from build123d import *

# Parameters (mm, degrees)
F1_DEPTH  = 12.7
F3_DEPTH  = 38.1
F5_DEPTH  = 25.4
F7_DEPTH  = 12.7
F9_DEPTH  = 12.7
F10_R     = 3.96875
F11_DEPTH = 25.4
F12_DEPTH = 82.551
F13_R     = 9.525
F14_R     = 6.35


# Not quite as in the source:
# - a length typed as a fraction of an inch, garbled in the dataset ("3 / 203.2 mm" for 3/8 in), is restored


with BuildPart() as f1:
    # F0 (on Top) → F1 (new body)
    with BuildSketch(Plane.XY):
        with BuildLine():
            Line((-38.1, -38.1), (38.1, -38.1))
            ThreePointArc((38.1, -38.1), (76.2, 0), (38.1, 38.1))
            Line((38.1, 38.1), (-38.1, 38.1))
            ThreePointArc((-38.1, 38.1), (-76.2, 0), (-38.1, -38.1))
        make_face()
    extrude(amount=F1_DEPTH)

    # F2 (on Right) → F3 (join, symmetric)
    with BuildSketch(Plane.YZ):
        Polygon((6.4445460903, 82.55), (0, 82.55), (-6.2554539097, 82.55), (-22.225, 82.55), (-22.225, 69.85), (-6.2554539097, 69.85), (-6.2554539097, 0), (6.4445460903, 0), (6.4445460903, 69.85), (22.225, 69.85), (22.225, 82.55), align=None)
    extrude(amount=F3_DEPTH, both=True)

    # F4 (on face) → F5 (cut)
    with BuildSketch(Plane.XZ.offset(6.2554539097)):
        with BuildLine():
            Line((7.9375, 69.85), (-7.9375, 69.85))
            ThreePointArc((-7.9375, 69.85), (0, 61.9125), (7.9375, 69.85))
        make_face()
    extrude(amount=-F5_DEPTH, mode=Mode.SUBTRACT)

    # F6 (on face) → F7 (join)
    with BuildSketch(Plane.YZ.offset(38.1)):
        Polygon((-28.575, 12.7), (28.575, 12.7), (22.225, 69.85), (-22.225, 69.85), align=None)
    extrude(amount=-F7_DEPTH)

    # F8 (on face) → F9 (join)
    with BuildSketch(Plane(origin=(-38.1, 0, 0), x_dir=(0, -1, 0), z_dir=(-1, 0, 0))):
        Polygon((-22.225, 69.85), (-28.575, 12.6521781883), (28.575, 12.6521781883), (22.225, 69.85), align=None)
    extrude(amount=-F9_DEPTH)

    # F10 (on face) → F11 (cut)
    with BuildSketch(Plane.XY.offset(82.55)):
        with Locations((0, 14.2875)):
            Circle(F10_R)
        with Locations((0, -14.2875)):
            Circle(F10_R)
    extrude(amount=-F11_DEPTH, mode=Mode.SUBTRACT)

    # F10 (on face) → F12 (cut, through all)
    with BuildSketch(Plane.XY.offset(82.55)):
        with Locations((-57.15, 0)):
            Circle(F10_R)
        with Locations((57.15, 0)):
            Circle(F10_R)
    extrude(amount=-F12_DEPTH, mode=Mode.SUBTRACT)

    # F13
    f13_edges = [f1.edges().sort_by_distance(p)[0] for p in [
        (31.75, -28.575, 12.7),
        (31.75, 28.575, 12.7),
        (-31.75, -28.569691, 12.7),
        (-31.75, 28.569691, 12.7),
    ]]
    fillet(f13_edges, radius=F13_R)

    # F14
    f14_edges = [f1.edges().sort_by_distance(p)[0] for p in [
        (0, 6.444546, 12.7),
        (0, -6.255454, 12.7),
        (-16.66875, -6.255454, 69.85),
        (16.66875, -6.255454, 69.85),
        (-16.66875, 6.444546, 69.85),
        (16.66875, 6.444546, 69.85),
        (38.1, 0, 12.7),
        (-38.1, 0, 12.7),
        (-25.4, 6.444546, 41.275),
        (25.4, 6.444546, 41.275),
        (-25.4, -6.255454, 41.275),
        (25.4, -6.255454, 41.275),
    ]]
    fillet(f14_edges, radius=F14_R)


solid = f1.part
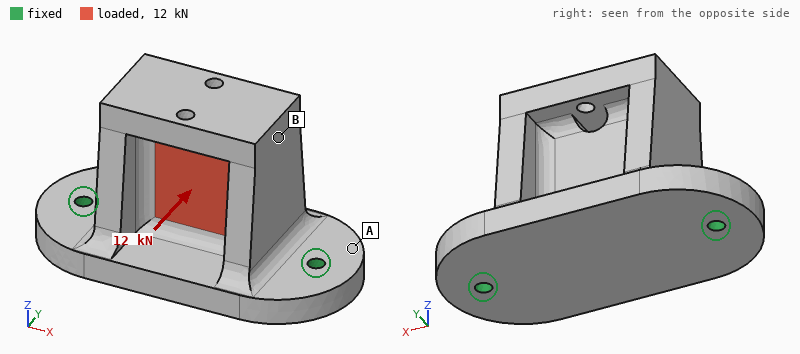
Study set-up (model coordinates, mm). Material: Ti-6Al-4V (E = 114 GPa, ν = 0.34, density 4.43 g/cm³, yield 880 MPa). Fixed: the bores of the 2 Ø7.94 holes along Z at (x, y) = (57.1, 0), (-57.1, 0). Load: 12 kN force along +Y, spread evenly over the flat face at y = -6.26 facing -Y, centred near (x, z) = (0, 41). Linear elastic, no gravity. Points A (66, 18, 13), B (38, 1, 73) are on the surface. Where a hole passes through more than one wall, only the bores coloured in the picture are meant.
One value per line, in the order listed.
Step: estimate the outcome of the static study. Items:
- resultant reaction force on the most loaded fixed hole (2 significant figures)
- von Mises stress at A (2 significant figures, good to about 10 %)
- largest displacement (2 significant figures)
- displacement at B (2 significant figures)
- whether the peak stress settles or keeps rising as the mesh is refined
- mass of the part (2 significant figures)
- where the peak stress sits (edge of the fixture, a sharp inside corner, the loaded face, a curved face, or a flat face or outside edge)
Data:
6.0 kN
53 MPa
0.24 mm
0.20 mm
keeps rising
1.3 kg
edge of the fixture
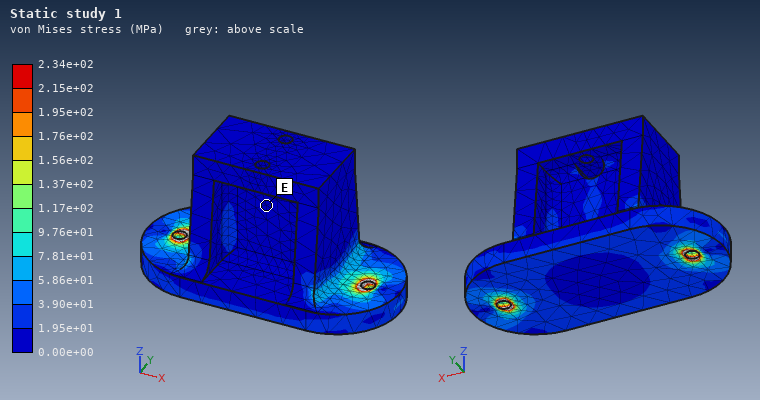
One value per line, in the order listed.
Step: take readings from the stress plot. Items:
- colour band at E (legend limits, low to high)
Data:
0.00e+00 to 1.95e+01 MPa
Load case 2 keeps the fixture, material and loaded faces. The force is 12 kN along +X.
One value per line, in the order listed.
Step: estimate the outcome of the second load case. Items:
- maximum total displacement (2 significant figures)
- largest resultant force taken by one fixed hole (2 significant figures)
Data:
32 µm
7.3 kN
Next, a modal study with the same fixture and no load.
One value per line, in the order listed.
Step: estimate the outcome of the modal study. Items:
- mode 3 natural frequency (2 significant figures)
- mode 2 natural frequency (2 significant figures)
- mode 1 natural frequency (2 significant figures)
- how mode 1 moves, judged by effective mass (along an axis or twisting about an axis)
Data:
3800 Hz
3700 Hz
1300 Hz
along Y
